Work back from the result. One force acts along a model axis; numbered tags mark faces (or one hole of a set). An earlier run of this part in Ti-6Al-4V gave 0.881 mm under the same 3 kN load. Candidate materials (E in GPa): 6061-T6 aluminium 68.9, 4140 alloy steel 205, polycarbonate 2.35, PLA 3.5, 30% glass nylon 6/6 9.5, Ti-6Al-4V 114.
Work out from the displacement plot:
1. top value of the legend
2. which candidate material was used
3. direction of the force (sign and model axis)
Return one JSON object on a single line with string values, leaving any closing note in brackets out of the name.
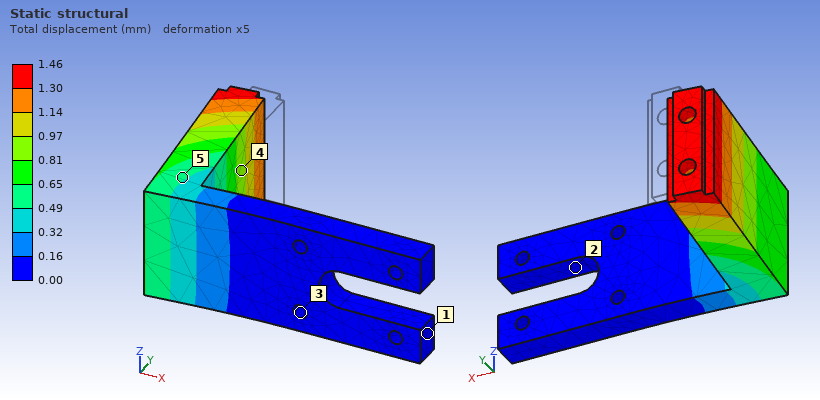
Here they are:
{"top value of the legend": "1.46 mm", "which candidate material was used": "6061-T6 aluminium", "direction of the force": "-X"}
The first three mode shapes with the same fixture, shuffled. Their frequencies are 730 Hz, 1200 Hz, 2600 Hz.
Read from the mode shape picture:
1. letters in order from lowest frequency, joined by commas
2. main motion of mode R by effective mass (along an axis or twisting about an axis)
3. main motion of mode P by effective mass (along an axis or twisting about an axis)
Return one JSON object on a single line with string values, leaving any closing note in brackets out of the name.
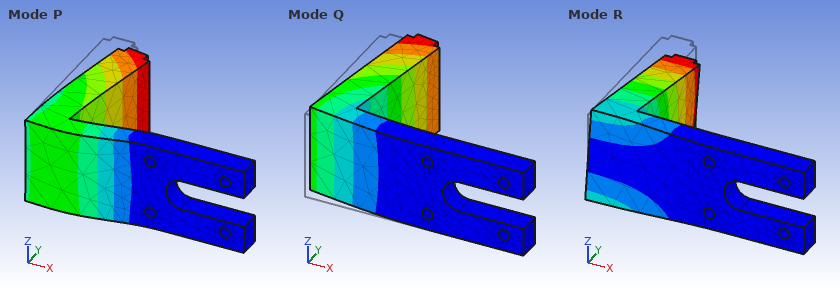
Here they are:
{"letters in order from lowest frequency, joined by commas": "Q, R, P", "main motion of mode R by effective mass": "along Z", "main motion of mode P by effective mass": "along Y"}
